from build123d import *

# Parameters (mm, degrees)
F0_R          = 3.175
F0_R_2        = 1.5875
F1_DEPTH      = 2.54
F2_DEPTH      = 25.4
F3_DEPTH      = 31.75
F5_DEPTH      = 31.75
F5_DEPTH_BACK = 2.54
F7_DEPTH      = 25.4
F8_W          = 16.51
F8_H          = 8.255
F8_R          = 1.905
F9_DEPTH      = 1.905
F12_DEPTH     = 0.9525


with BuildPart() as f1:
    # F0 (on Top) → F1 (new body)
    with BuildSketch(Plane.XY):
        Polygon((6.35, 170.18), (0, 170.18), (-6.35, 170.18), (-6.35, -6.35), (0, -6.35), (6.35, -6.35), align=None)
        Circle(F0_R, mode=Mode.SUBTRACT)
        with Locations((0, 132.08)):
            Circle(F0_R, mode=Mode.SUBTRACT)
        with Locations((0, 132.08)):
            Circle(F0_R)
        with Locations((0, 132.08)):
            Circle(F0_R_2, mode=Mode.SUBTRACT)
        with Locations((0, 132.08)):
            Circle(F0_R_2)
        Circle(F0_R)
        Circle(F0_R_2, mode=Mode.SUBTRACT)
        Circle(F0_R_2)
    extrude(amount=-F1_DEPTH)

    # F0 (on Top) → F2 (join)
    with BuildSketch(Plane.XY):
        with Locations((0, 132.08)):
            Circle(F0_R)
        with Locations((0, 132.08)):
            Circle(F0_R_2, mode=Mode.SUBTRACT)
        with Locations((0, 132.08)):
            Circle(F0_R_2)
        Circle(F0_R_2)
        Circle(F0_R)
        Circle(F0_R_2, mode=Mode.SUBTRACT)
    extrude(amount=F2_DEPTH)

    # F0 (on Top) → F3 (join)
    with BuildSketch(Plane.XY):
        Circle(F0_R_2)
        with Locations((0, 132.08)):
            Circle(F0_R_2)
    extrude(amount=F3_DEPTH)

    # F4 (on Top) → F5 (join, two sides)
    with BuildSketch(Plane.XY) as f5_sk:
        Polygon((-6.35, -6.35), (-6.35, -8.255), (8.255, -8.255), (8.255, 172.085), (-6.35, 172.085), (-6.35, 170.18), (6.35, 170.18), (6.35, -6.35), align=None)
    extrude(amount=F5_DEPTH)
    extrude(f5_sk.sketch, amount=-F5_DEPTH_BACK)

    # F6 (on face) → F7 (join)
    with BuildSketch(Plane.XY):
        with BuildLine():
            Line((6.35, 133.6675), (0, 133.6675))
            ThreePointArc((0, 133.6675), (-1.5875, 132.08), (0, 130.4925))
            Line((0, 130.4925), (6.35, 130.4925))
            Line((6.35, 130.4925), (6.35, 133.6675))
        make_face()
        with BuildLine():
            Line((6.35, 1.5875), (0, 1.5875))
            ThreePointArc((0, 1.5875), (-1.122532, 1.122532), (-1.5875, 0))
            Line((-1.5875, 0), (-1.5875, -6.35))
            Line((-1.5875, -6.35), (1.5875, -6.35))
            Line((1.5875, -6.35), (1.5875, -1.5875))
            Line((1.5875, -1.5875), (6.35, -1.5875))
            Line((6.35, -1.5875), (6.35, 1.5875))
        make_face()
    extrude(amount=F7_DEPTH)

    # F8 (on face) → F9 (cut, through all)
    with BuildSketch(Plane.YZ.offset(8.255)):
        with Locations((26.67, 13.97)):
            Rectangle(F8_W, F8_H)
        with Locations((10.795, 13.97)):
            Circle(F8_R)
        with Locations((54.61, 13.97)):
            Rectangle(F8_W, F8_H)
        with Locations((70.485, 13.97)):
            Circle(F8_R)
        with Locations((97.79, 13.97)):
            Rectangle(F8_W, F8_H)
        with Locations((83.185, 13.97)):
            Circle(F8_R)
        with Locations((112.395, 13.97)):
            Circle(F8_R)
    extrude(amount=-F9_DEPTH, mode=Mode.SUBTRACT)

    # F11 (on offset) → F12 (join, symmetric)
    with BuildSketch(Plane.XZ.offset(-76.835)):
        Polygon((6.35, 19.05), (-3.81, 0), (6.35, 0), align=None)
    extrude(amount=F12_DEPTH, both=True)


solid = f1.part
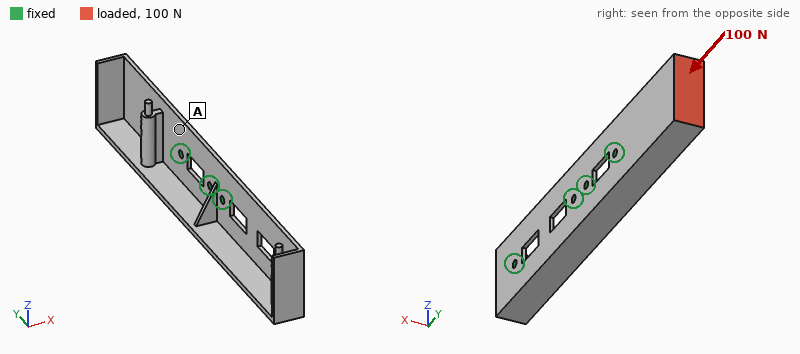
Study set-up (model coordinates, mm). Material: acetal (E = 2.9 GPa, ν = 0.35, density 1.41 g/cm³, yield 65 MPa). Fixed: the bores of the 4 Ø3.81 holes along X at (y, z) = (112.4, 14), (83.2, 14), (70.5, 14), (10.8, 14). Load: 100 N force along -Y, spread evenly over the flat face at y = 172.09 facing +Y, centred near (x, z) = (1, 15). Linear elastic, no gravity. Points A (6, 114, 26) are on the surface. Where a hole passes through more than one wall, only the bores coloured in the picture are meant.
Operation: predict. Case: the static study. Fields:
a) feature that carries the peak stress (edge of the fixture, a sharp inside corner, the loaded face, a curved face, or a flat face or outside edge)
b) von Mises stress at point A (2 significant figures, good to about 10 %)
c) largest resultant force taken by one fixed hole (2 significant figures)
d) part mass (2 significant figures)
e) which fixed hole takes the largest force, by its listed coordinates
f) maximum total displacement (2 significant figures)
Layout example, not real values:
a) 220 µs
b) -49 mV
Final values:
a) the loaded face
b) 2.3 MPa
c) 46 N
d) 30 g
e) (112.4, 14)
f) 1.9 mm
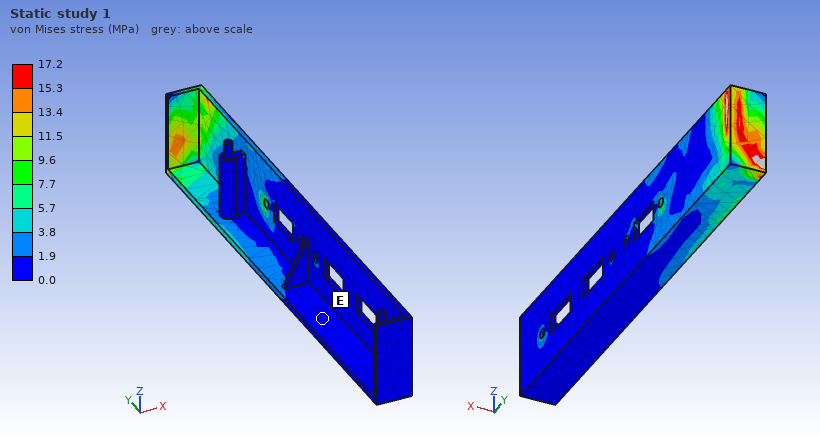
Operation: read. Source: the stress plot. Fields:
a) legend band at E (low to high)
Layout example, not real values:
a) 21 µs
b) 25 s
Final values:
a) 0.0 to 1.9 MPa
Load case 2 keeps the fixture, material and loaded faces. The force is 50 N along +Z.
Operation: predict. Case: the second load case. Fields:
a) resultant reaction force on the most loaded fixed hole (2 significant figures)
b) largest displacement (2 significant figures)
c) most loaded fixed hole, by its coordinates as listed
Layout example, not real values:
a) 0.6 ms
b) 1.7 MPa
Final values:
a) 110 N
b) 2.2 mm
c) (112.4, 14)
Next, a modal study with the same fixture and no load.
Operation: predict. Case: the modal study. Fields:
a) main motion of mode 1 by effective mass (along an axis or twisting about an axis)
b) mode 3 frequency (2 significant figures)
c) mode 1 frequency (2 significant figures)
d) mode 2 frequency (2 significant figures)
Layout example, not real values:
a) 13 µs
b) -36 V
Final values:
a) along X
b) 570 Hz
c) 270 Hz
d) 360 Hz
